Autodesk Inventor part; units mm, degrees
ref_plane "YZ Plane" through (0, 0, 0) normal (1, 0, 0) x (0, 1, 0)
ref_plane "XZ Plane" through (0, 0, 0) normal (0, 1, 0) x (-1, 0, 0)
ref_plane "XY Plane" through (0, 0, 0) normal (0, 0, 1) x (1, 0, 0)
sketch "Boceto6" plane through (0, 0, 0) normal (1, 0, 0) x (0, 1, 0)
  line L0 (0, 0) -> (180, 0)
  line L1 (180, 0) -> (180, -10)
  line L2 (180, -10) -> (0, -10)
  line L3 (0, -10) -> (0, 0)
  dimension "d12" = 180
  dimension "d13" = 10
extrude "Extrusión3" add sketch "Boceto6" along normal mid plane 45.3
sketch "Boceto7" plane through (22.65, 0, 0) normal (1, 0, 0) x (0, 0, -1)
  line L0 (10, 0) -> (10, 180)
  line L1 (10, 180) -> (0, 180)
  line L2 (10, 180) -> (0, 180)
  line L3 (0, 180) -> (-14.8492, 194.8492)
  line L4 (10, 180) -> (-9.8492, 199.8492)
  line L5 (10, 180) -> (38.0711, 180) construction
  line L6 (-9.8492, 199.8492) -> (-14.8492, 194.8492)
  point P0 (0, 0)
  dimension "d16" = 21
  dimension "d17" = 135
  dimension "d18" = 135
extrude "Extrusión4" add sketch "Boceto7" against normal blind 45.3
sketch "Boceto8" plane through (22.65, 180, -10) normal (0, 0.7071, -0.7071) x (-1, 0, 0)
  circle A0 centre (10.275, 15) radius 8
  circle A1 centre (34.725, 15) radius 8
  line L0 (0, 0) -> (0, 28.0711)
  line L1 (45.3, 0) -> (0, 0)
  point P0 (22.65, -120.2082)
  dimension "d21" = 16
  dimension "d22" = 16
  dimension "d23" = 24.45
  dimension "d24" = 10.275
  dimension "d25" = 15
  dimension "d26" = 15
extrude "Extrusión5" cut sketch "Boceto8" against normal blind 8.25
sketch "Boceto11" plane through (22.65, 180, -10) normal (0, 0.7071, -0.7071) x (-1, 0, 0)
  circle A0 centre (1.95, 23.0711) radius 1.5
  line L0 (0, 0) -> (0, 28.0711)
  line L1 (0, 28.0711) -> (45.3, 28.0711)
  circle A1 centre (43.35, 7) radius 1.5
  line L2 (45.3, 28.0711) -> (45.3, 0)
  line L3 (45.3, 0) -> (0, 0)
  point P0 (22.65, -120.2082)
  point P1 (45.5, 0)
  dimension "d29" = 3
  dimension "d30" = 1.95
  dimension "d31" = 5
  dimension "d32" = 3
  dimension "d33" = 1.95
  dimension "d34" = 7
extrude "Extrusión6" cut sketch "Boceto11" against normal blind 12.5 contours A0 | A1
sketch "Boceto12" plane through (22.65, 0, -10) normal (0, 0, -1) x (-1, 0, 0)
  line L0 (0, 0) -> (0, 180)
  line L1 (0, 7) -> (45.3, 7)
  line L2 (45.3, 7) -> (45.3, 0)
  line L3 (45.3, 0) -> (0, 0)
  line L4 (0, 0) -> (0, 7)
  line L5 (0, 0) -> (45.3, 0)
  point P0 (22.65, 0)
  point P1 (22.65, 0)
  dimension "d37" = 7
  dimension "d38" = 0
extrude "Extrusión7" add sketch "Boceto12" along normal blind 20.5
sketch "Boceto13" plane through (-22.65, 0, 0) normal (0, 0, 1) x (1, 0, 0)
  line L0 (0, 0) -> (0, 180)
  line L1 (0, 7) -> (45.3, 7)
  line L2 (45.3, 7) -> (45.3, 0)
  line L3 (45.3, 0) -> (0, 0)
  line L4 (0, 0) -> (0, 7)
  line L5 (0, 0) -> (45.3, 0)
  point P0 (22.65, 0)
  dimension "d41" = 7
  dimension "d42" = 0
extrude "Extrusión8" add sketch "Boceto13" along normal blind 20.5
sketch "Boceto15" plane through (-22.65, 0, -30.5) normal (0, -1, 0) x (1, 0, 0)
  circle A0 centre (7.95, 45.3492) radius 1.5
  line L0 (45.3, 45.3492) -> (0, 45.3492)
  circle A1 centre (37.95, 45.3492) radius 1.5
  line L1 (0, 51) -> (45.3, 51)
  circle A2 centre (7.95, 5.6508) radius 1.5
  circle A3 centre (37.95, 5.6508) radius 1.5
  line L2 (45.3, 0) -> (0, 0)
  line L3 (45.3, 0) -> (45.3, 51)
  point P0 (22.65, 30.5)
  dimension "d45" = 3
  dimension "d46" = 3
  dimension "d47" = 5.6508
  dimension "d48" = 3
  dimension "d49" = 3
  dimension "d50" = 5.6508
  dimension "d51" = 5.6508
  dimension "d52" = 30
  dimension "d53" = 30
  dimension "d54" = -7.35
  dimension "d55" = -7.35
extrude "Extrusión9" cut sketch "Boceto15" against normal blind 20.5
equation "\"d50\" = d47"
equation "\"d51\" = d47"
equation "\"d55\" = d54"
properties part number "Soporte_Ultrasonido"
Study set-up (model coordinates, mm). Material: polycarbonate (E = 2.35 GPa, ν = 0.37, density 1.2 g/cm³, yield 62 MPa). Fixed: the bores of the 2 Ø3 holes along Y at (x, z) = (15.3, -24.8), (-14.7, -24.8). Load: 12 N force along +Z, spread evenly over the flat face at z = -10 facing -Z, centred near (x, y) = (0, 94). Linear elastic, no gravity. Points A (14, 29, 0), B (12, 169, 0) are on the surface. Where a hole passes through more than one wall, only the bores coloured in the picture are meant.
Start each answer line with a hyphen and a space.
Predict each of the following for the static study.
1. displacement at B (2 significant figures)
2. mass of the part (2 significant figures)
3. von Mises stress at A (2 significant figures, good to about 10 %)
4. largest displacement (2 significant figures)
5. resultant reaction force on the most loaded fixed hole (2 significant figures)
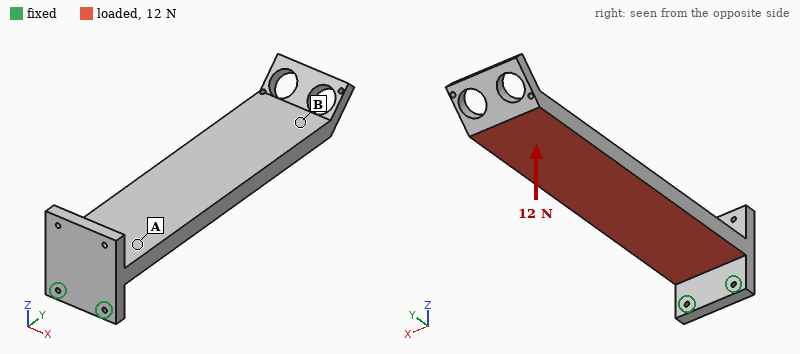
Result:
- 2.0 mm
- 120 g
- 1.0 MPa
- 2.4 mm
- 7.2 N
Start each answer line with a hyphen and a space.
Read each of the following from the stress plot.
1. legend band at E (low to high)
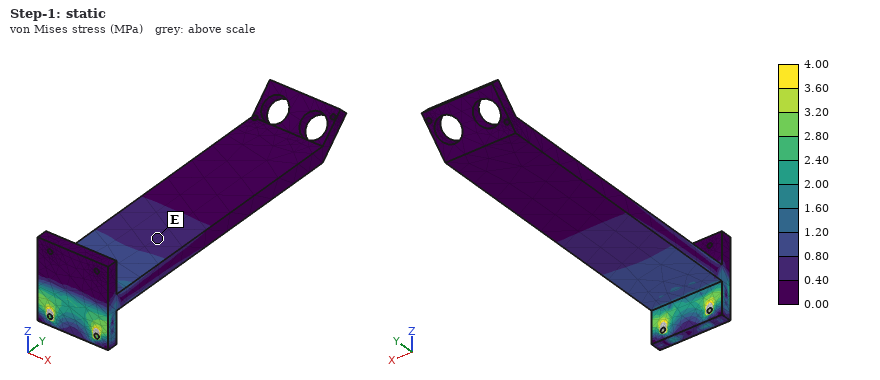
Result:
- 0.40 to 0.80 MPa
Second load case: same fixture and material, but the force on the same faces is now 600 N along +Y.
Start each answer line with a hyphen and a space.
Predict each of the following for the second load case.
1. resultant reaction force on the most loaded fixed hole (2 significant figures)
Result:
- 300 N
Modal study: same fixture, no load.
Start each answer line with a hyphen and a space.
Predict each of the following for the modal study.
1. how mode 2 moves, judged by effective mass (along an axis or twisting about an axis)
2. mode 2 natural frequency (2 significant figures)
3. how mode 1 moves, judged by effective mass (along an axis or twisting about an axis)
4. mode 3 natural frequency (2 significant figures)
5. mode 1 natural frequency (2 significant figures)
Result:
- along X
- 110 Hz
- along Z
- 300 Hz
- 43 Hz
